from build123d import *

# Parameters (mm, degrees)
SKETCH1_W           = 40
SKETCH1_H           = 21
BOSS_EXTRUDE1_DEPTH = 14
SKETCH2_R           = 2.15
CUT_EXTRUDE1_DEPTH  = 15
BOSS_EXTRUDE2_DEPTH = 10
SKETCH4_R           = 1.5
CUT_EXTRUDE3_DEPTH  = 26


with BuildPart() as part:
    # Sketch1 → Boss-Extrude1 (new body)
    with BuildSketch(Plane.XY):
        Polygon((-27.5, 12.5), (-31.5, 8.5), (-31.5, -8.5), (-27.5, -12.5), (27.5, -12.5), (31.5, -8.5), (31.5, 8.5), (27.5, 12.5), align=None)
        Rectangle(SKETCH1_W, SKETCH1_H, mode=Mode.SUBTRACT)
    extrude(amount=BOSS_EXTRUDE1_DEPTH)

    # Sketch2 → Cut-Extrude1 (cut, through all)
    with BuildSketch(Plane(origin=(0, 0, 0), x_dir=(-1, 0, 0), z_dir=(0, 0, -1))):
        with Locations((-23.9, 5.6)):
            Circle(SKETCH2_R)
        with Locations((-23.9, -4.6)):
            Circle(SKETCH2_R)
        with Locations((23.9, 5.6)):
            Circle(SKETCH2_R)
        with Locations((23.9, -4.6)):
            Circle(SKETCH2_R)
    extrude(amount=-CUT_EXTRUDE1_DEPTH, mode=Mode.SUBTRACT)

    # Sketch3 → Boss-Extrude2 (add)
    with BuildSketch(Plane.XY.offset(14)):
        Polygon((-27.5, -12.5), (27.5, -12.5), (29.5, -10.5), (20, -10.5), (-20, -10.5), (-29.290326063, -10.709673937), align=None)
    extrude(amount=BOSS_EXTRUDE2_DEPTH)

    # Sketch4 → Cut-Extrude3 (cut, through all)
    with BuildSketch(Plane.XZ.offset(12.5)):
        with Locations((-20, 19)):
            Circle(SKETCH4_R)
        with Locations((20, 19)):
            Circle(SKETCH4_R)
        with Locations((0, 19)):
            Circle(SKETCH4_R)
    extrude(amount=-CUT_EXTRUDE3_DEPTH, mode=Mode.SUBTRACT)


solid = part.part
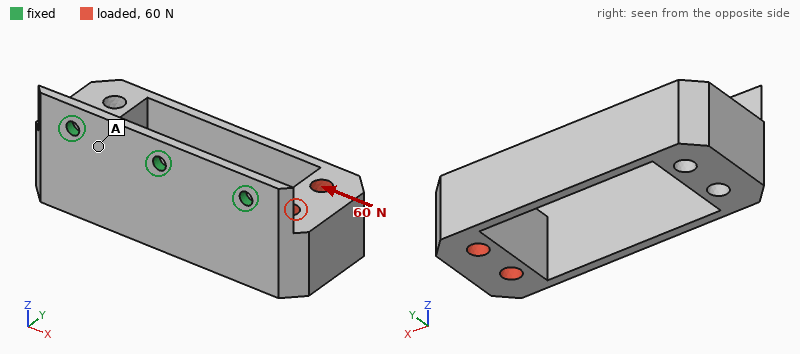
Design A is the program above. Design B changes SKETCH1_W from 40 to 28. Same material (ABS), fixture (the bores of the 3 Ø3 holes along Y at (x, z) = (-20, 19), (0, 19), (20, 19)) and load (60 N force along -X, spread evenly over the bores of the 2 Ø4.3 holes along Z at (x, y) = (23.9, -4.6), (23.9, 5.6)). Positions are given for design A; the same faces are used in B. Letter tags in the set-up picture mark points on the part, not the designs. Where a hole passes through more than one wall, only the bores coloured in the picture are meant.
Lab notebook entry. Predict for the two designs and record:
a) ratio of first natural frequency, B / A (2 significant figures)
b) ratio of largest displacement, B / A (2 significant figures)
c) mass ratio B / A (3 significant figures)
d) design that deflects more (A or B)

0.94
0.42
1.35
A
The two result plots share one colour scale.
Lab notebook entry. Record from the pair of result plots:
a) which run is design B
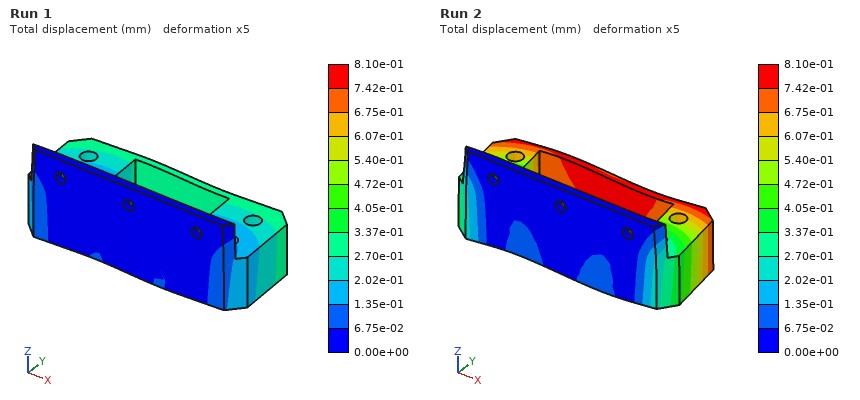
Run 1
